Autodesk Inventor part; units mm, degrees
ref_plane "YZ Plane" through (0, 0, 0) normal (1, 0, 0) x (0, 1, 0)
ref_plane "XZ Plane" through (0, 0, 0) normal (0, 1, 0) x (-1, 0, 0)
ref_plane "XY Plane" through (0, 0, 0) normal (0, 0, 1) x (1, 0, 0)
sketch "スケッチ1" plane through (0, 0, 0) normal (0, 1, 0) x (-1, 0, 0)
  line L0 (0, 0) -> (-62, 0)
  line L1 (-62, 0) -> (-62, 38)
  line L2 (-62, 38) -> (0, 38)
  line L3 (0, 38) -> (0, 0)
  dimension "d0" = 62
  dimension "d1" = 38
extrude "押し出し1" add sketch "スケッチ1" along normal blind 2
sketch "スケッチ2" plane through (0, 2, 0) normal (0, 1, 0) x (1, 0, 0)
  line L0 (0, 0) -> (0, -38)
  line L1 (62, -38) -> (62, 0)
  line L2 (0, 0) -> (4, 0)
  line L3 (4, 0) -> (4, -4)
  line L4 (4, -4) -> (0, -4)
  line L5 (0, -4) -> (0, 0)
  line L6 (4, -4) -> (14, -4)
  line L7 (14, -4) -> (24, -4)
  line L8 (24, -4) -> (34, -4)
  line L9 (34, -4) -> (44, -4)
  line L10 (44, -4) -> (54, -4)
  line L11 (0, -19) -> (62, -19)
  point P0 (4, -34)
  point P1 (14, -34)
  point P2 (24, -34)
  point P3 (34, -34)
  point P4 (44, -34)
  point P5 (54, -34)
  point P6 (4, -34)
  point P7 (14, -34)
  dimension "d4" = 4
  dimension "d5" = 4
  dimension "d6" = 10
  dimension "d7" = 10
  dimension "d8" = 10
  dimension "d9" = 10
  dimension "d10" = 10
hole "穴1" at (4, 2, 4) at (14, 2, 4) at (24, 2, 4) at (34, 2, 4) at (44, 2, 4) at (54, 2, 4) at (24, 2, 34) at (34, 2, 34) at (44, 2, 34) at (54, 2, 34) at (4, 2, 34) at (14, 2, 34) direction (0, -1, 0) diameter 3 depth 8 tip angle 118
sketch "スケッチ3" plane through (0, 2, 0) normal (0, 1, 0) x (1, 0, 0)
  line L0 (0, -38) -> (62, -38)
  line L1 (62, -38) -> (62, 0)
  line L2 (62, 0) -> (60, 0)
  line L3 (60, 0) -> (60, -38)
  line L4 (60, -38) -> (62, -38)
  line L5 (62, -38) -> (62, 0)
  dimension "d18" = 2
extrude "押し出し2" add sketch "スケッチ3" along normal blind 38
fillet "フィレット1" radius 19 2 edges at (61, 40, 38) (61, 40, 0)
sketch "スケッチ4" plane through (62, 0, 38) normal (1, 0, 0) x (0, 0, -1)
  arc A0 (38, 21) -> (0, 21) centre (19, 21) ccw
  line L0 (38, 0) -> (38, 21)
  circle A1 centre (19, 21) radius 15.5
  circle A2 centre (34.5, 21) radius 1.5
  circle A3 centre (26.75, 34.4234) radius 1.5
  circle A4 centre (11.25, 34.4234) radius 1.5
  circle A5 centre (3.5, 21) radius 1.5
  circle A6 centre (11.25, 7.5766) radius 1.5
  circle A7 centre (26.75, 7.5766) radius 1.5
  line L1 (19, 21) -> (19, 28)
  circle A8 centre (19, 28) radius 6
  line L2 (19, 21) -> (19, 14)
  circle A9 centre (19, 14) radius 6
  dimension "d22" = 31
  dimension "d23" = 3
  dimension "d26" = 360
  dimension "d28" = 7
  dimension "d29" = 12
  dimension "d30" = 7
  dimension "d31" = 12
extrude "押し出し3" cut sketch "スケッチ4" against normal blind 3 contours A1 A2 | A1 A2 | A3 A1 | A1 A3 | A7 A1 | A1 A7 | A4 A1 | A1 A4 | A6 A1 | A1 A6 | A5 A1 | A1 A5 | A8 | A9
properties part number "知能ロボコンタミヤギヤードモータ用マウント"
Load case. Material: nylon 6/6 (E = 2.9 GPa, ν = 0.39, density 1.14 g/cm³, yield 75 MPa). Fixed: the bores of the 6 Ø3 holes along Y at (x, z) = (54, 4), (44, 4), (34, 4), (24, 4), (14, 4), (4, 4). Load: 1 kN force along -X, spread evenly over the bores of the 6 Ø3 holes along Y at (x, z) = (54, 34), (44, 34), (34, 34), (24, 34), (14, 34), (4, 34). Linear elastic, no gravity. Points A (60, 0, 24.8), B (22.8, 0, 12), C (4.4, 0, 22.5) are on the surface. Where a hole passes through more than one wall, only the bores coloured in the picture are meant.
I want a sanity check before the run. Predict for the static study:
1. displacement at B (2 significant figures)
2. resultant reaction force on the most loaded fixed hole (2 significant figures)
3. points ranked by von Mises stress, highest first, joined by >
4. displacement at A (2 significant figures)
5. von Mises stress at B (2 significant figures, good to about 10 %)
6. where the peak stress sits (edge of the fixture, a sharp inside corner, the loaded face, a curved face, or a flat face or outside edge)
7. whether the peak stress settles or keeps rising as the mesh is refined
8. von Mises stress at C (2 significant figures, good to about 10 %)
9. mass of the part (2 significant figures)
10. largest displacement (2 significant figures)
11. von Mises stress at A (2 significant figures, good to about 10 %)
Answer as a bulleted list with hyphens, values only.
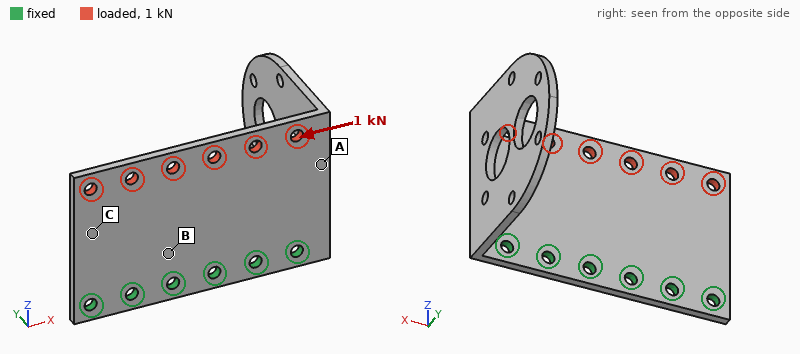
- 0.075 mm
- 520 N
- B > C > A
- 0.30 mm
- 18 MPa
- edge of the fixture
- keeps rising
- 11 MPa
- 7.5 g
- 0.48 mm
- 5.3 MPa
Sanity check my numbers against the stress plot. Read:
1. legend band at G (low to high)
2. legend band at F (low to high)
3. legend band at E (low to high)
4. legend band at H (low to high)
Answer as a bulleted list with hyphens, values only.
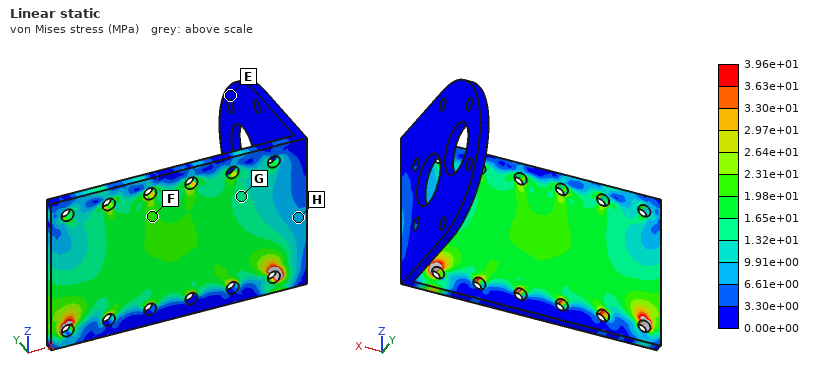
- 1.32e+01 to 1.65e+01 MPa
- 1.98e+01 to 2.31e+01 MPa
- 0.00e+00 to 3.30e+00 MPa
- 6.61e+00 to 9.91e+00 MPa
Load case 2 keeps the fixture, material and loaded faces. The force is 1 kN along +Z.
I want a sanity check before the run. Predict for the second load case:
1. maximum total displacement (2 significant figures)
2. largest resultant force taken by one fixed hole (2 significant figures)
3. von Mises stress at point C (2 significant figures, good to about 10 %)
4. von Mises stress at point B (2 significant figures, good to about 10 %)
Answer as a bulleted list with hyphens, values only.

- 0.12 mm
- 200 N
- 8.7 MPa
- 7.9 MPa
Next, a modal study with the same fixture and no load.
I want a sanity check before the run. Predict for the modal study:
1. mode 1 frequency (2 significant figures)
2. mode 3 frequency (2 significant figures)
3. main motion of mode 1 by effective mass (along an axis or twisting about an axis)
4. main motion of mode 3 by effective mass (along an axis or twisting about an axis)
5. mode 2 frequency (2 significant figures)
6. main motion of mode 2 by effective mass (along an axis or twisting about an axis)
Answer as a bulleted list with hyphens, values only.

- 280 Hz
- 620 Hz
- along X
- along Y
- 380 Hz
- along Y
